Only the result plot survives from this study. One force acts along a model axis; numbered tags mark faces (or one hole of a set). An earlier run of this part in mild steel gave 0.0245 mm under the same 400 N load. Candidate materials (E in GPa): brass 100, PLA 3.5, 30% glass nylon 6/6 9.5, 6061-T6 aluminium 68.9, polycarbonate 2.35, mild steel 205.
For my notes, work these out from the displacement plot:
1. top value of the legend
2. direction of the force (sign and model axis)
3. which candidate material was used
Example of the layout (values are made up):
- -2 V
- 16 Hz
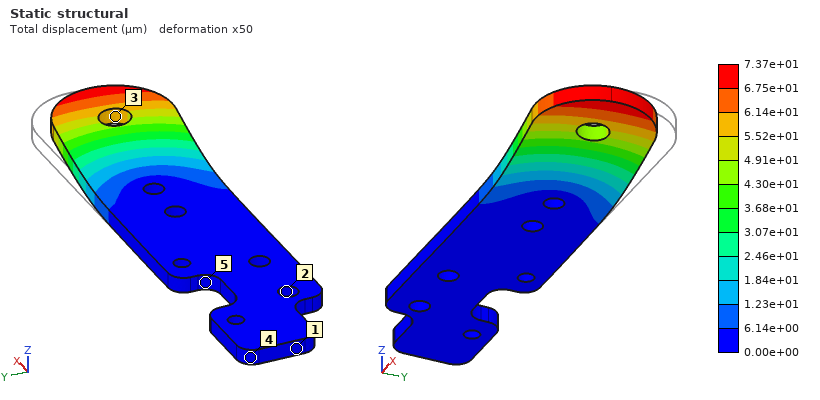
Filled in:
- 7.37e+01 µm
- -Y
- 6061-T6 aluminium
